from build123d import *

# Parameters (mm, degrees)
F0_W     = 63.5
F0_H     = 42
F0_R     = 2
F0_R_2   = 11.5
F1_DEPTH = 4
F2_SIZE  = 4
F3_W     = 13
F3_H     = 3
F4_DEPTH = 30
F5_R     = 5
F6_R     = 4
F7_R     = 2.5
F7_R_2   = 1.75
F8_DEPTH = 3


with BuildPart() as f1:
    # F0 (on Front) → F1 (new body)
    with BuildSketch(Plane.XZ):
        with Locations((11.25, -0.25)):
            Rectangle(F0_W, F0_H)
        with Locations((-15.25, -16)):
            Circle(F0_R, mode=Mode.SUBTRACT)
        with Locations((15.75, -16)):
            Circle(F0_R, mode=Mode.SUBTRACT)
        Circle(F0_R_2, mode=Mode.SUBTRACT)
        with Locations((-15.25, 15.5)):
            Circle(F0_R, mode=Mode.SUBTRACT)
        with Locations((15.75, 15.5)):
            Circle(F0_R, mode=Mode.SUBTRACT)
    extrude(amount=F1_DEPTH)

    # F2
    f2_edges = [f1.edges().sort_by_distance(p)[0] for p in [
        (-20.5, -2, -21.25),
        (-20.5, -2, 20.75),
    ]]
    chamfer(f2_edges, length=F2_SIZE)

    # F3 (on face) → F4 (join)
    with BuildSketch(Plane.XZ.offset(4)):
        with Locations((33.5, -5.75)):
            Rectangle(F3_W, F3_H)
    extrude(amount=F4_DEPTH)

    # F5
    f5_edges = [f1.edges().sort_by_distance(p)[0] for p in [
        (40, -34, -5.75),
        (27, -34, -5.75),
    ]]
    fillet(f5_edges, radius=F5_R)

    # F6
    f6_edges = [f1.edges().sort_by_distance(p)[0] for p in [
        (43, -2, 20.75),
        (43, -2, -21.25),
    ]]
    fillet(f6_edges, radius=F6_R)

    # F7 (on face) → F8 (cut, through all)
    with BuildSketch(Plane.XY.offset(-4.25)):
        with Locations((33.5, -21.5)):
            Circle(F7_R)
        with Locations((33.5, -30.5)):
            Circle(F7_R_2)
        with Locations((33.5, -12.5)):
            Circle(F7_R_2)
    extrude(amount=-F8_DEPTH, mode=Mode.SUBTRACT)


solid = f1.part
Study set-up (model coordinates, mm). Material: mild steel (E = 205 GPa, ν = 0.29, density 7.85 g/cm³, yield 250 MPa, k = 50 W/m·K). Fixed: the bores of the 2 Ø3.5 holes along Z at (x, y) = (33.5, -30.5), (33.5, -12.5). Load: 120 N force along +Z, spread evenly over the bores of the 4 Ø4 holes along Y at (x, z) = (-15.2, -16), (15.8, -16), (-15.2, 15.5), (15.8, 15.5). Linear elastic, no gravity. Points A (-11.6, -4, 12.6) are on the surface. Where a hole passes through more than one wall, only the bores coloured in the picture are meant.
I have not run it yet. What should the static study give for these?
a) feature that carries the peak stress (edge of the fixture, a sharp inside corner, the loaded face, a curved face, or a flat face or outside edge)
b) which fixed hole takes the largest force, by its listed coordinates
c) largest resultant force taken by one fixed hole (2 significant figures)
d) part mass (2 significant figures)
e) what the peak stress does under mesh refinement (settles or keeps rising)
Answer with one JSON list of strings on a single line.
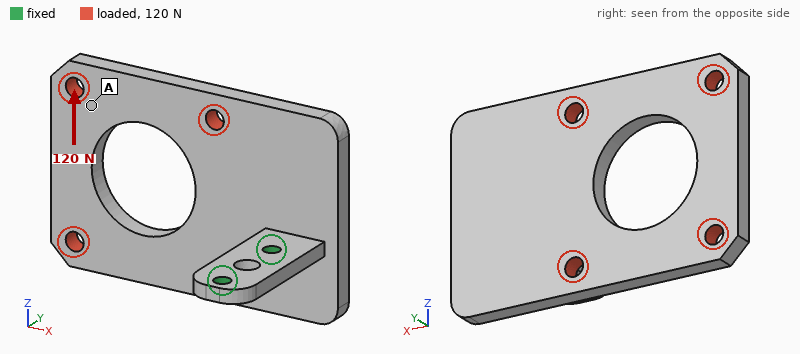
["edge of the fixture", "(33.5, -12.5)", "130 N", "76 g", "keeps rising"]
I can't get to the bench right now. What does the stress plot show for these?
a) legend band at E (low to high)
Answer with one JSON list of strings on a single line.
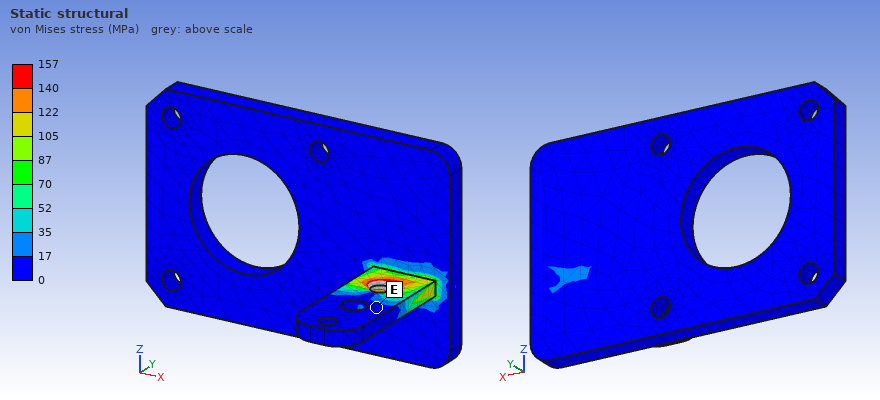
["0 to 17 MPa"]
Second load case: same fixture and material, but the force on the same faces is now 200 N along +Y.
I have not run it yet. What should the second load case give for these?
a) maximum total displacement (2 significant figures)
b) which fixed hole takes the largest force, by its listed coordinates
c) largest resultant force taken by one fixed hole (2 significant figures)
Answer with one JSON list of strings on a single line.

["0.23 mm", "(33.5, -12.5)", "260 N"]
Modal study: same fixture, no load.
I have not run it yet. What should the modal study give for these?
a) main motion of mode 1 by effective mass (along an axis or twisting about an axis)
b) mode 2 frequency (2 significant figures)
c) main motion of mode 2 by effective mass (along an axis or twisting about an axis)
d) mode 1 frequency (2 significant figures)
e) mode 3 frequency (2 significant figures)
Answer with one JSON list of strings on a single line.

["along Z", "930 Hz", "along Y", "690 Hz", "1200 Hz"]
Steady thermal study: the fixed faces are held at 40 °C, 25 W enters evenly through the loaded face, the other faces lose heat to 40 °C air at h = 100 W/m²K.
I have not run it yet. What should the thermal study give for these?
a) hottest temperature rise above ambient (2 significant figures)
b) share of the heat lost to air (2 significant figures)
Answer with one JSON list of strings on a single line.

["69 K", "85 %"]
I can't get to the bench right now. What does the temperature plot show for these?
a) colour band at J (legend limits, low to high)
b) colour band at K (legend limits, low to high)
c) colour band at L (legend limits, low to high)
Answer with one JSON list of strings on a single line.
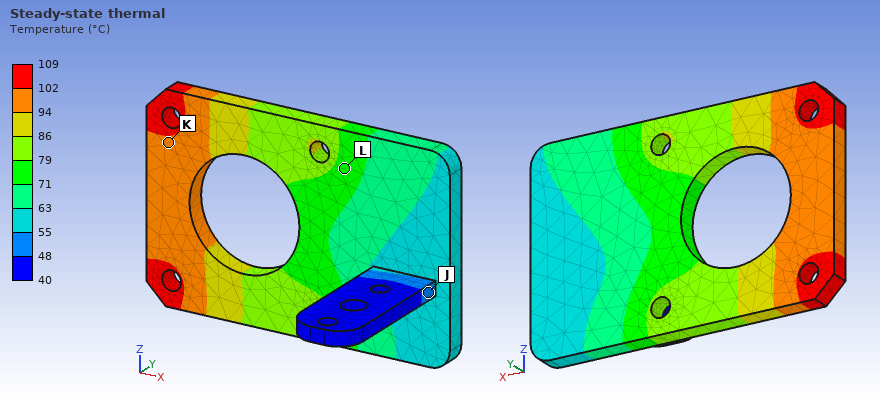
["48 to 55 °C", "94 to 102 °C", "71 to 79 °C"]
